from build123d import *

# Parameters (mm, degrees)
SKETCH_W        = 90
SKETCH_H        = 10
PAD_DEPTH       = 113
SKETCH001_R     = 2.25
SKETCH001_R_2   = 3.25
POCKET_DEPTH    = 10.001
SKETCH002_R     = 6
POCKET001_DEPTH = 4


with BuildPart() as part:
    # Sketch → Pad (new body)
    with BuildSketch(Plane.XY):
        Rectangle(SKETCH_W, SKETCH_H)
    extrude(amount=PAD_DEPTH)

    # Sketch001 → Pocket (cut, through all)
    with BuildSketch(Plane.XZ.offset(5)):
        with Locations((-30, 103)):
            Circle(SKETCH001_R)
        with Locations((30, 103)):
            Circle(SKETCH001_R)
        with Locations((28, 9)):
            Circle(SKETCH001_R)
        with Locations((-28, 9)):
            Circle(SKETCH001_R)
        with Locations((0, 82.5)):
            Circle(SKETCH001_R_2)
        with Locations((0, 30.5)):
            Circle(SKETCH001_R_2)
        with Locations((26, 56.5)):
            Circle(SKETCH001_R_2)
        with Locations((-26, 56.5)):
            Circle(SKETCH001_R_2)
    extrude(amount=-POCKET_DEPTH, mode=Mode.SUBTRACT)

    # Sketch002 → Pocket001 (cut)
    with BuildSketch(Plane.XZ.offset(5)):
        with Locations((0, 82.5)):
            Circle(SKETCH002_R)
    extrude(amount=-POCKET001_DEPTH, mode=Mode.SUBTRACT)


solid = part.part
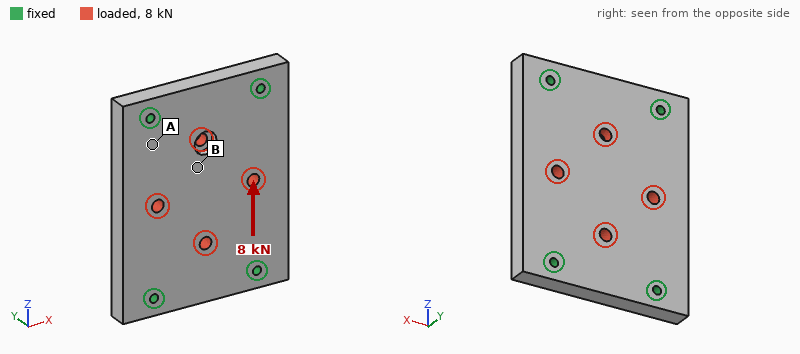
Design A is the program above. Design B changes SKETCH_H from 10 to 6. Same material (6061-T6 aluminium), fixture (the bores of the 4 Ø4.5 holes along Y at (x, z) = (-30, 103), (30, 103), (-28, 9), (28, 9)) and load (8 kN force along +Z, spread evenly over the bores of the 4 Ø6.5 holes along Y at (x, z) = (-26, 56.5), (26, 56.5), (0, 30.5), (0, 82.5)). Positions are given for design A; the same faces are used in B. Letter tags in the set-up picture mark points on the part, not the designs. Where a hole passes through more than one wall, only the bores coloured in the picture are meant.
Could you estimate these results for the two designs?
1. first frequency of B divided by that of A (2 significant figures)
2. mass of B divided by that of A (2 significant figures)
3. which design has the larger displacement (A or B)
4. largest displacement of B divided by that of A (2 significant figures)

0.66
0.60
B
1.7
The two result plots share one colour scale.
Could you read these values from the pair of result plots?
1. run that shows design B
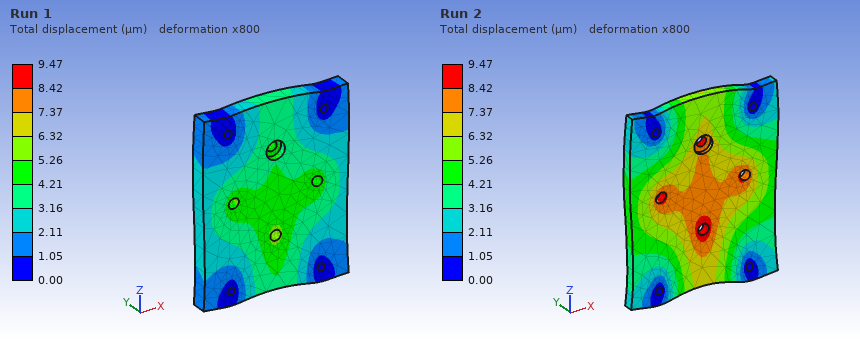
Run 2
